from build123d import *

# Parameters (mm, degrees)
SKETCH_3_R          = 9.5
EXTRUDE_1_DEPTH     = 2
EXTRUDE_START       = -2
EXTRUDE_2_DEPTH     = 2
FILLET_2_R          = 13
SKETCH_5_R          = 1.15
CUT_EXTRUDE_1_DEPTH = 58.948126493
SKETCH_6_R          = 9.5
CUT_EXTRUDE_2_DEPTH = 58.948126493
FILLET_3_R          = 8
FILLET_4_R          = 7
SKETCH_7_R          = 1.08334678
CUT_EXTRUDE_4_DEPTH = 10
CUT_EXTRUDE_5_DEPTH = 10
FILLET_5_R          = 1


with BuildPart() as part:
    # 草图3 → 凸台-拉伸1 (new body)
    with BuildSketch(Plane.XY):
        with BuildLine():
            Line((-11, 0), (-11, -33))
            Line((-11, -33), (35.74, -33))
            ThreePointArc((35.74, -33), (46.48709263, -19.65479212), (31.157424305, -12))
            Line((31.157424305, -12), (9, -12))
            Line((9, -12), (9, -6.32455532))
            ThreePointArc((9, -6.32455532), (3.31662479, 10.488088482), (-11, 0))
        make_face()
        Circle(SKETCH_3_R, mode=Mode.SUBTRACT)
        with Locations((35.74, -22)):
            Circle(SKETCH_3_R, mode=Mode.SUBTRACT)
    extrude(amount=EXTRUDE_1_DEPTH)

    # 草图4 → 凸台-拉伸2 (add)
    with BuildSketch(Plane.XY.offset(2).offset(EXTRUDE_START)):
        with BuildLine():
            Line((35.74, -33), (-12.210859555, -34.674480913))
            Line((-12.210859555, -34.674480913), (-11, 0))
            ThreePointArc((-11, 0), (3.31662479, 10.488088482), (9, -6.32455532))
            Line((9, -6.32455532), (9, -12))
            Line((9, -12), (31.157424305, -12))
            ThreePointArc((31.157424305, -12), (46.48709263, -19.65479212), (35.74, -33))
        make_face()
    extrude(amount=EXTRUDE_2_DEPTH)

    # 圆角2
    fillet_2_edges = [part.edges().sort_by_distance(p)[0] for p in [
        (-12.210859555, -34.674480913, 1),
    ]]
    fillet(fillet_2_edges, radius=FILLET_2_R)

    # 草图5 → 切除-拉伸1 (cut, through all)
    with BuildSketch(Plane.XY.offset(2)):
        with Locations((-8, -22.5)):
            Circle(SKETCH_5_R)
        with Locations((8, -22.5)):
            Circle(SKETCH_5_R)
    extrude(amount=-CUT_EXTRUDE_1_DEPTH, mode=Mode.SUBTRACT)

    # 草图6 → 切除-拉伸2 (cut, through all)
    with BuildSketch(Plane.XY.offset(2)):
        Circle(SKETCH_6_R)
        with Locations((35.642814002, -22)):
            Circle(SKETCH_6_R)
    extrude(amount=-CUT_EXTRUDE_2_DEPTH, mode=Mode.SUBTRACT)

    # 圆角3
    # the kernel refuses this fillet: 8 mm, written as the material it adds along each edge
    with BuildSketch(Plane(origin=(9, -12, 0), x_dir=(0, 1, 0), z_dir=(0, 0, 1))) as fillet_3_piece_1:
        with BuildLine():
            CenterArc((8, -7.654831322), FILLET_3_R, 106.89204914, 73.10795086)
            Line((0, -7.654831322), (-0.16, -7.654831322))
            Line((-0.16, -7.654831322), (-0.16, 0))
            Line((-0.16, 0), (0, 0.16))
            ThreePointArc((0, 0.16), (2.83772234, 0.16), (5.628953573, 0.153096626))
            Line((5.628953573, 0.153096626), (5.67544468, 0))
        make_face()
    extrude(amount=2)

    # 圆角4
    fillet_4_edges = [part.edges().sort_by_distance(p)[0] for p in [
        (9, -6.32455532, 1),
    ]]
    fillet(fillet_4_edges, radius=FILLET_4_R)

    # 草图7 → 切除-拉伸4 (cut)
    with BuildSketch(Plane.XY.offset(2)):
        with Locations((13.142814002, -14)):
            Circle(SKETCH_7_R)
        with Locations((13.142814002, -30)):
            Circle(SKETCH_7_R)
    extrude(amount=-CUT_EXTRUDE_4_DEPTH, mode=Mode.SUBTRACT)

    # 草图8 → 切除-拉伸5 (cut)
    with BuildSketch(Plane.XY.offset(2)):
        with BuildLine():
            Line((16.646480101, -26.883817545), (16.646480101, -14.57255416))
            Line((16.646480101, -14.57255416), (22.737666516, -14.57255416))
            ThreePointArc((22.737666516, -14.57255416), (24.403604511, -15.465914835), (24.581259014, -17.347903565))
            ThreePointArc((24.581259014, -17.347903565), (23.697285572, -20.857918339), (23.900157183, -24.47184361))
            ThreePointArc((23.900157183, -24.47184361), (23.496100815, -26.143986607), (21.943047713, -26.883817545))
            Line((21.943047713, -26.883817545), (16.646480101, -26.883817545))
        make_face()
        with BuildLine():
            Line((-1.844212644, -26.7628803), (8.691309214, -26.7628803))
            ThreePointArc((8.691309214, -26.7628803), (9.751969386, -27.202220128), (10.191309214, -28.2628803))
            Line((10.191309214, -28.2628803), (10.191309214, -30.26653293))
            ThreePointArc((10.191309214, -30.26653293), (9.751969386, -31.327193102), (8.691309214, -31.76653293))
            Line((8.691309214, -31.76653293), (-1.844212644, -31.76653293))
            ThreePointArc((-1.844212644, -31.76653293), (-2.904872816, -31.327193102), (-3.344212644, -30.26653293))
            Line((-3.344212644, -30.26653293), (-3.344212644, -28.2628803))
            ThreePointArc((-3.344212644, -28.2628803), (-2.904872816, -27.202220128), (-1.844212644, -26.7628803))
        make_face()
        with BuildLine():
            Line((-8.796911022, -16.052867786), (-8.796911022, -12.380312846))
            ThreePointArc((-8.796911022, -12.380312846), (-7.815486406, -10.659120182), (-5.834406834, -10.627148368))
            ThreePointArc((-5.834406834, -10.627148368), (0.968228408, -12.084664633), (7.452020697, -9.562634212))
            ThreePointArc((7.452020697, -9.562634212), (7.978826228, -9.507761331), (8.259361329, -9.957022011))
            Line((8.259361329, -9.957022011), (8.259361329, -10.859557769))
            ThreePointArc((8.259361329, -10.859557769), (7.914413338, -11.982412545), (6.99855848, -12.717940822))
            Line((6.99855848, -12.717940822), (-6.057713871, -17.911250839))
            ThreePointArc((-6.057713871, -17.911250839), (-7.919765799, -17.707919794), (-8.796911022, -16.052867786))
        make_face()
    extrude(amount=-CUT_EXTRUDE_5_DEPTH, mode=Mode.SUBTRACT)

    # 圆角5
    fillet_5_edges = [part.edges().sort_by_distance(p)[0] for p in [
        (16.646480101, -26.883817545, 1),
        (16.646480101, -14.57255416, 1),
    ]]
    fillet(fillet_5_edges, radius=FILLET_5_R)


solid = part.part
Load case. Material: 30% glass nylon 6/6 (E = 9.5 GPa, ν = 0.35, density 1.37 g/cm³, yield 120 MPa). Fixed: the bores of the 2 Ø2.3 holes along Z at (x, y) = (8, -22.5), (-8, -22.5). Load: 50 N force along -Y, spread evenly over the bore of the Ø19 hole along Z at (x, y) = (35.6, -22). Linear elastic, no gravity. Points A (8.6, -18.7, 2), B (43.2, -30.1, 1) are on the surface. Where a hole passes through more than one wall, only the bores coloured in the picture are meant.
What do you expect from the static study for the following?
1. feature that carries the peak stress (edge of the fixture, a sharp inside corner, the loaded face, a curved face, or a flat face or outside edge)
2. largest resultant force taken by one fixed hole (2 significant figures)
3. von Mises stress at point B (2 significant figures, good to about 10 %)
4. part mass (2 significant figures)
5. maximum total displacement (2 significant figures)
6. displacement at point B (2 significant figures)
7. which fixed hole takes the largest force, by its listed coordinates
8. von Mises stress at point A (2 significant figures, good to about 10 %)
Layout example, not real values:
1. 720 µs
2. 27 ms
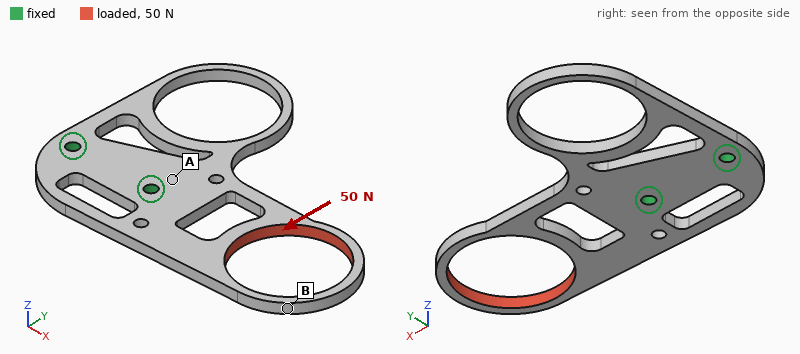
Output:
1. a curved face
2. 120 N
3. 40 MPa
4. 2.3 g
5. 0.67 mm
6. 0.64 mm
7. (8, -22.5)
8. 8.0 MPa
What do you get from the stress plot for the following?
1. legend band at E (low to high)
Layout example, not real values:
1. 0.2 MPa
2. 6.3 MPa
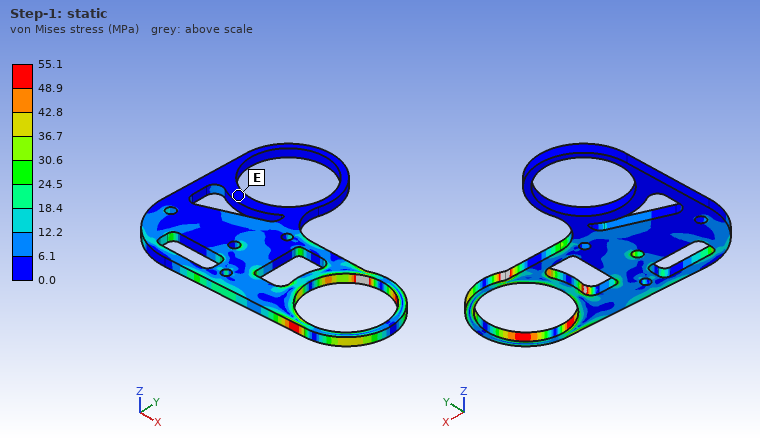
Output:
1. 0.0 to 6.1 MPa
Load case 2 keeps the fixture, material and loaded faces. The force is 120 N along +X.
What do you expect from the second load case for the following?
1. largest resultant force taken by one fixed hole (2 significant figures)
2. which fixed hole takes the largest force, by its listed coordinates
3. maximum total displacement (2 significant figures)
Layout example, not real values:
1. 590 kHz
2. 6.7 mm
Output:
1. 90 N
2. (8, -22.5)
3. 0.19 mm
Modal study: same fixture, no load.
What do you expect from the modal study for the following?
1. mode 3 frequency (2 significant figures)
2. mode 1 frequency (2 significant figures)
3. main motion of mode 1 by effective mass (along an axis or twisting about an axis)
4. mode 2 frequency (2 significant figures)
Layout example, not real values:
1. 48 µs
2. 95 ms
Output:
1. 1800 Hz
2. 800 Hz
3. along Z
4. 1100 Hz
